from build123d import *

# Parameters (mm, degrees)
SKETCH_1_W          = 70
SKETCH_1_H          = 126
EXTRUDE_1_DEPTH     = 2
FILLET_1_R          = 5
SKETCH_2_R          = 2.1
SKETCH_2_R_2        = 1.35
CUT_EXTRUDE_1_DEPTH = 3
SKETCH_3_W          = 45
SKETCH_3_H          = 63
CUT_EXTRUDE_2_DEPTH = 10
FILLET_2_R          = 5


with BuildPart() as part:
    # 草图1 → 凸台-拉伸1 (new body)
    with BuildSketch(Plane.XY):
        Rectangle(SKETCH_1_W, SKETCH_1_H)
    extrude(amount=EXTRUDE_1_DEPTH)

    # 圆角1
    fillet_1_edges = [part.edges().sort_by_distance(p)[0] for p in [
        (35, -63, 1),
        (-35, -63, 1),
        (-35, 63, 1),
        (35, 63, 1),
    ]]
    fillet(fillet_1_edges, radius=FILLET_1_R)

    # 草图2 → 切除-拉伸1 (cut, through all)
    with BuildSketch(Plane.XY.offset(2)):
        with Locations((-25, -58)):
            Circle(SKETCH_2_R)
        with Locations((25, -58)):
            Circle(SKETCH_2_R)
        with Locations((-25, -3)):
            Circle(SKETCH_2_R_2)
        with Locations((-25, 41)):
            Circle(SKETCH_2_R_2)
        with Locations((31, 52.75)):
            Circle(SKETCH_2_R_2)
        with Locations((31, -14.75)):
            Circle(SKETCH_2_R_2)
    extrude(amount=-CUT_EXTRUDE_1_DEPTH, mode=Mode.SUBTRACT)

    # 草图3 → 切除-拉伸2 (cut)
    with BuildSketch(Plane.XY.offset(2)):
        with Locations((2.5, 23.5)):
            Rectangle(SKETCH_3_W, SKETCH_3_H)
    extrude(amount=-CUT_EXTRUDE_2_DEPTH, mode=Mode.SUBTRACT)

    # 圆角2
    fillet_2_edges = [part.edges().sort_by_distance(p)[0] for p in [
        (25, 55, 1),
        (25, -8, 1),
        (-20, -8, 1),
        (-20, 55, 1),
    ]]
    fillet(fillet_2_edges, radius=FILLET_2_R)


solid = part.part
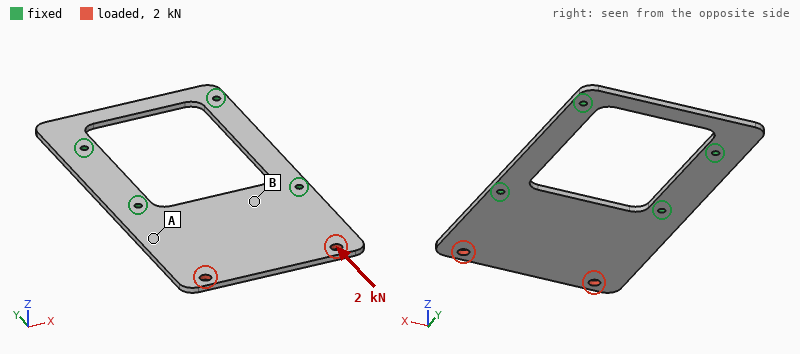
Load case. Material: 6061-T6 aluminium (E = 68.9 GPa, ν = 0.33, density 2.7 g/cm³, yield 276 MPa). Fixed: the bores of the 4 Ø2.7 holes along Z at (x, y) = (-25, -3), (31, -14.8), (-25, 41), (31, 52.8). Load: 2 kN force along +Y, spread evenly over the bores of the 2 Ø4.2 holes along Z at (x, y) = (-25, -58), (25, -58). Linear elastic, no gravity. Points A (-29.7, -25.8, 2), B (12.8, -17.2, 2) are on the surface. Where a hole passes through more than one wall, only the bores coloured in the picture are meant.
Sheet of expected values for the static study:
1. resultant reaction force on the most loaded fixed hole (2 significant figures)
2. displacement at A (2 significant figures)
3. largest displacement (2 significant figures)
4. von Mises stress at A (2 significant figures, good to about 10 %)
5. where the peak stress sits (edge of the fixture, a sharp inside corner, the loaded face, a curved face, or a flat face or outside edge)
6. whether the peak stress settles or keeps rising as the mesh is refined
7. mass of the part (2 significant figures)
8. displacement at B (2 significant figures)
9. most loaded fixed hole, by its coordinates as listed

1.0 kN
11 µm
28 µm
25 MPa
edge of the fixture
keeps rising
32 g
11 µm
(-25, -3)
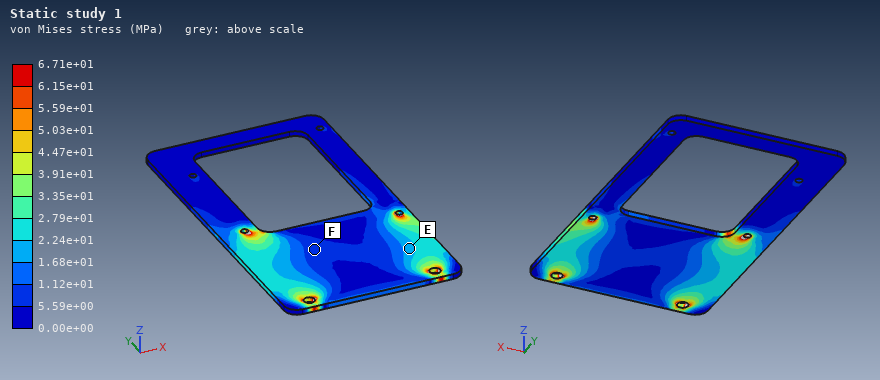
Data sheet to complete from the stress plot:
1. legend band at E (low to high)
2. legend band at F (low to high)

1.68e+01 to 2.24e+01 MPa
5.59e+00 to 1.12e+01 MPa
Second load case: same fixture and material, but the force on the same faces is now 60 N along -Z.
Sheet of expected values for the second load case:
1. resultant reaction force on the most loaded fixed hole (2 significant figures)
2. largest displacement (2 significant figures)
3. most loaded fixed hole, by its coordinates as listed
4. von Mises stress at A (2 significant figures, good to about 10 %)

40 N
1.4 mm
(31, -14.8)
39 MPa
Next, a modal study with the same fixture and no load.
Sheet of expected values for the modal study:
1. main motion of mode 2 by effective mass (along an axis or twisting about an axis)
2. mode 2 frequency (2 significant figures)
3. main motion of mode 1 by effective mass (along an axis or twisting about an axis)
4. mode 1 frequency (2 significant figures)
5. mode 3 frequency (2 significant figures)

twisting about Y
1200 Hz
along Z
440 Hz
2300 Hz
